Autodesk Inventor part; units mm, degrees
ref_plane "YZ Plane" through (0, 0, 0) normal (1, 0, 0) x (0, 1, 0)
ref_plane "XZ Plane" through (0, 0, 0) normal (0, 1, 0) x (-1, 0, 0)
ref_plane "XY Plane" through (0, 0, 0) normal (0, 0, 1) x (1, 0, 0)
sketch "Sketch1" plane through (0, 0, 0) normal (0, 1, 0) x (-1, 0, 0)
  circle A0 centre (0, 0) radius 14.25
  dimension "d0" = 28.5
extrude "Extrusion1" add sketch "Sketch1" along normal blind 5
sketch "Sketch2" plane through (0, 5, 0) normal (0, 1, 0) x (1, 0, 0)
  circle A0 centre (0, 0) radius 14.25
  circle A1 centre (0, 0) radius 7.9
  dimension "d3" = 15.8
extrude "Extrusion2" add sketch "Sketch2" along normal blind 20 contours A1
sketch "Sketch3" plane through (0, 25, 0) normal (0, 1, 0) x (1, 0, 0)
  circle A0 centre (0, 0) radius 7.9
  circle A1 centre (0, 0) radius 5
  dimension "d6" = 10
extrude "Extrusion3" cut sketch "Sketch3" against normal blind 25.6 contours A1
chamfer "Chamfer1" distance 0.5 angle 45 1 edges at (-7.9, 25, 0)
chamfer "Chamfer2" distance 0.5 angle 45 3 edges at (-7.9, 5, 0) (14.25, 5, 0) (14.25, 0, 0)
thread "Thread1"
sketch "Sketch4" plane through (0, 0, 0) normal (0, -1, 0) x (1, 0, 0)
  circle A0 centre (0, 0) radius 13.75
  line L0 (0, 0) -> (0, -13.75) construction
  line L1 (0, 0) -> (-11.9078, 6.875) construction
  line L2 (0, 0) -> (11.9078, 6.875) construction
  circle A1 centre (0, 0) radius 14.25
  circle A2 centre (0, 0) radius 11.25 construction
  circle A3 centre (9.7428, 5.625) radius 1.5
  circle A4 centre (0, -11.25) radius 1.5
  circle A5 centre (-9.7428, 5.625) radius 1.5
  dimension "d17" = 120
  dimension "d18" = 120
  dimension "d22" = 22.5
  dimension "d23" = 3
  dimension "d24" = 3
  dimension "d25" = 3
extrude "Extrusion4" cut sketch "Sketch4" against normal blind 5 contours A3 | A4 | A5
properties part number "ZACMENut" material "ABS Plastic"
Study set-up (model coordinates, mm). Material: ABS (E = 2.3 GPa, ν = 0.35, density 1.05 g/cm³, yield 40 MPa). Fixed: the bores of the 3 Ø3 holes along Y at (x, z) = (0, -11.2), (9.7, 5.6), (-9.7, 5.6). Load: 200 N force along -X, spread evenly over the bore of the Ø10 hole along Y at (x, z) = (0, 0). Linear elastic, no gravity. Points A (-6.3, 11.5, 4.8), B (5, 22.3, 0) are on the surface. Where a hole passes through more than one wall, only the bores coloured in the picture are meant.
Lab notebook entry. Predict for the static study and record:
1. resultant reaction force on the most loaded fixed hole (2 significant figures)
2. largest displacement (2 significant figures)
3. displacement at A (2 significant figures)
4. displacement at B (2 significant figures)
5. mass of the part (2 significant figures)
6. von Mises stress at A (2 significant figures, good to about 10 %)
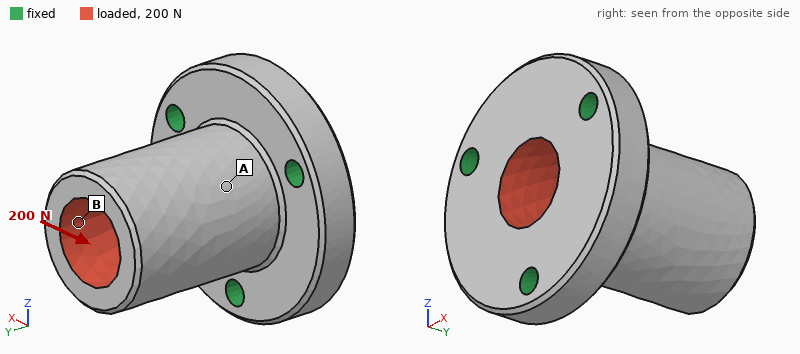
120 N
0.11 mm
0.044 mm
0.097 mm
5.3 g
2.3 MPa
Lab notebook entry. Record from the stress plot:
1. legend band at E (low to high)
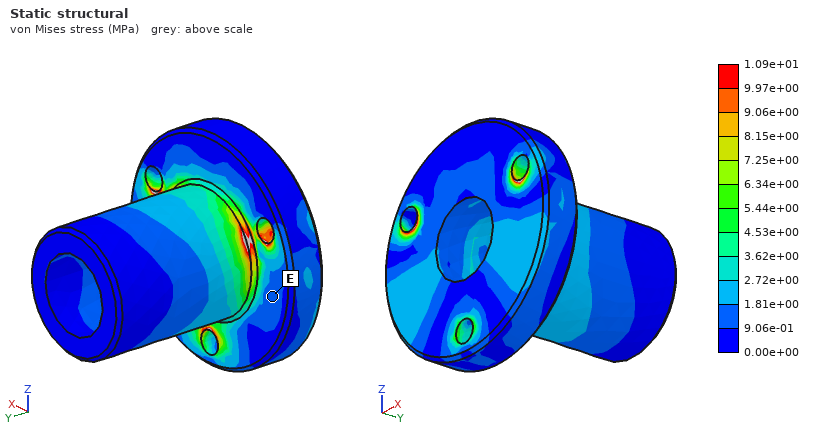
9.06e-01 to 1.81e+00 MPa
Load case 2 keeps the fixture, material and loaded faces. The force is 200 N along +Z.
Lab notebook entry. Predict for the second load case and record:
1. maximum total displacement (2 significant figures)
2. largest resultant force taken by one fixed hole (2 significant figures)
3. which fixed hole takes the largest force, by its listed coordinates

0.11 mm
130 N
(0, -11.2)
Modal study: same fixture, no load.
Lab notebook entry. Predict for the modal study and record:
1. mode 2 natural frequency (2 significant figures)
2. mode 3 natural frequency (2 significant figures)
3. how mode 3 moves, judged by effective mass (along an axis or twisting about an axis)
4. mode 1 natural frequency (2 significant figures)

4500 Hz
9700 Hz
along Y
4500 Hz
